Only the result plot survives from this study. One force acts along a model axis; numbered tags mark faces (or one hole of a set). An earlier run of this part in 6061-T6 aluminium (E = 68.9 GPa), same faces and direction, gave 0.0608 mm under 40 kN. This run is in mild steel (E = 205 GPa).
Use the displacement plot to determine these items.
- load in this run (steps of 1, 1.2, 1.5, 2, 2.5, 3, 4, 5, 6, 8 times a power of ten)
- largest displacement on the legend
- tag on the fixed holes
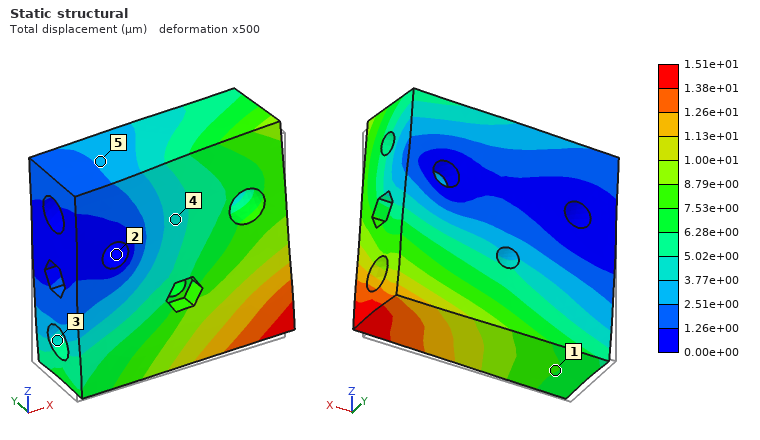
30 kN
1.51e+01 µm
2
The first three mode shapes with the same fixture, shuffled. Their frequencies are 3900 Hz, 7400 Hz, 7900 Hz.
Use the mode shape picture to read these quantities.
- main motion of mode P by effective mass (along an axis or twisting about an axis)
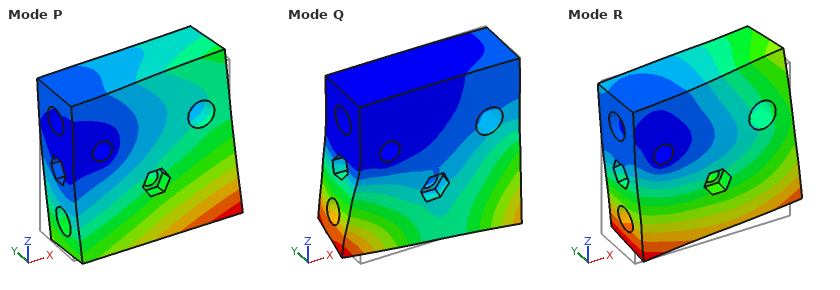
along Y
